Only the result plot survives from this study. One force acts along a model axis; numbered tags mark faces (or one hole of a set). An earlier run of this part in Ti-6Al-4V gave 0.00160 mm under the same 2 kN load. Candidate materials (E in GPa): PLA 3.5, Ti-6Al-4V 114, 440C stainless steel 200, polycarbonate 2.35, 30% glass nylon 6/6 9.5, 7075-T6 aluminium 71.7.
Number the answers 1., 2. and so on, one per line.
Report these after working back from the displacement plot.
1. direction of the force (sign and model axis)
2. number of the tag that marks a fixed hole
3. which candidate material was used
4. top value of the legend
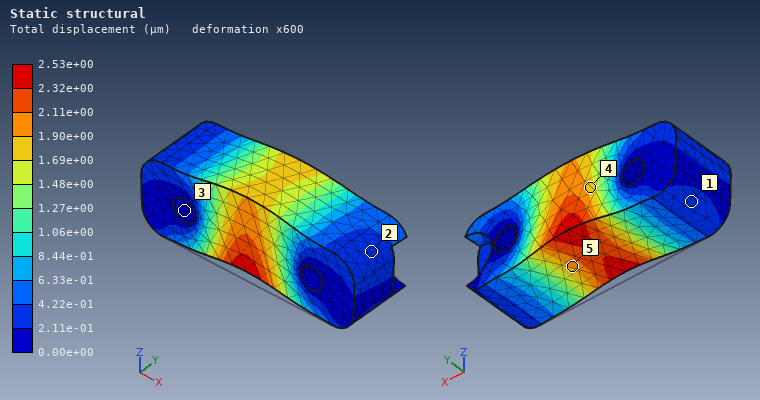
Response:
1. +Z
2. 3
3. 7075-T6 aluminium
4. 2.53e+00 µm
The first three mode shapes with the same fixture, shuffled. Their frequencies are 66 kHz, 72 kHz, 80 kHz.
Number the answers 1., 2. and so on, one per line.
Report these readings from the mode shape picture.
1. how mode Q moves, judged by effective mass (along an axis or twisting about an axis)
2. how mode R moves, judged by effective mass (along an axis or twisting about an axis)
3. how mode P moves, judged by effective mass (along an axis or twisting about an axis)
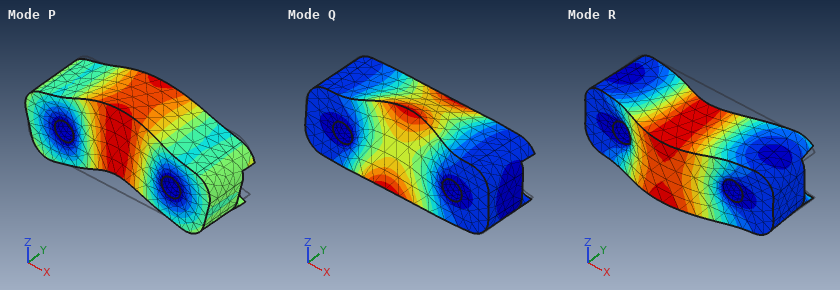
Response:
1. twisting about X
2. along Y
3. along Z
